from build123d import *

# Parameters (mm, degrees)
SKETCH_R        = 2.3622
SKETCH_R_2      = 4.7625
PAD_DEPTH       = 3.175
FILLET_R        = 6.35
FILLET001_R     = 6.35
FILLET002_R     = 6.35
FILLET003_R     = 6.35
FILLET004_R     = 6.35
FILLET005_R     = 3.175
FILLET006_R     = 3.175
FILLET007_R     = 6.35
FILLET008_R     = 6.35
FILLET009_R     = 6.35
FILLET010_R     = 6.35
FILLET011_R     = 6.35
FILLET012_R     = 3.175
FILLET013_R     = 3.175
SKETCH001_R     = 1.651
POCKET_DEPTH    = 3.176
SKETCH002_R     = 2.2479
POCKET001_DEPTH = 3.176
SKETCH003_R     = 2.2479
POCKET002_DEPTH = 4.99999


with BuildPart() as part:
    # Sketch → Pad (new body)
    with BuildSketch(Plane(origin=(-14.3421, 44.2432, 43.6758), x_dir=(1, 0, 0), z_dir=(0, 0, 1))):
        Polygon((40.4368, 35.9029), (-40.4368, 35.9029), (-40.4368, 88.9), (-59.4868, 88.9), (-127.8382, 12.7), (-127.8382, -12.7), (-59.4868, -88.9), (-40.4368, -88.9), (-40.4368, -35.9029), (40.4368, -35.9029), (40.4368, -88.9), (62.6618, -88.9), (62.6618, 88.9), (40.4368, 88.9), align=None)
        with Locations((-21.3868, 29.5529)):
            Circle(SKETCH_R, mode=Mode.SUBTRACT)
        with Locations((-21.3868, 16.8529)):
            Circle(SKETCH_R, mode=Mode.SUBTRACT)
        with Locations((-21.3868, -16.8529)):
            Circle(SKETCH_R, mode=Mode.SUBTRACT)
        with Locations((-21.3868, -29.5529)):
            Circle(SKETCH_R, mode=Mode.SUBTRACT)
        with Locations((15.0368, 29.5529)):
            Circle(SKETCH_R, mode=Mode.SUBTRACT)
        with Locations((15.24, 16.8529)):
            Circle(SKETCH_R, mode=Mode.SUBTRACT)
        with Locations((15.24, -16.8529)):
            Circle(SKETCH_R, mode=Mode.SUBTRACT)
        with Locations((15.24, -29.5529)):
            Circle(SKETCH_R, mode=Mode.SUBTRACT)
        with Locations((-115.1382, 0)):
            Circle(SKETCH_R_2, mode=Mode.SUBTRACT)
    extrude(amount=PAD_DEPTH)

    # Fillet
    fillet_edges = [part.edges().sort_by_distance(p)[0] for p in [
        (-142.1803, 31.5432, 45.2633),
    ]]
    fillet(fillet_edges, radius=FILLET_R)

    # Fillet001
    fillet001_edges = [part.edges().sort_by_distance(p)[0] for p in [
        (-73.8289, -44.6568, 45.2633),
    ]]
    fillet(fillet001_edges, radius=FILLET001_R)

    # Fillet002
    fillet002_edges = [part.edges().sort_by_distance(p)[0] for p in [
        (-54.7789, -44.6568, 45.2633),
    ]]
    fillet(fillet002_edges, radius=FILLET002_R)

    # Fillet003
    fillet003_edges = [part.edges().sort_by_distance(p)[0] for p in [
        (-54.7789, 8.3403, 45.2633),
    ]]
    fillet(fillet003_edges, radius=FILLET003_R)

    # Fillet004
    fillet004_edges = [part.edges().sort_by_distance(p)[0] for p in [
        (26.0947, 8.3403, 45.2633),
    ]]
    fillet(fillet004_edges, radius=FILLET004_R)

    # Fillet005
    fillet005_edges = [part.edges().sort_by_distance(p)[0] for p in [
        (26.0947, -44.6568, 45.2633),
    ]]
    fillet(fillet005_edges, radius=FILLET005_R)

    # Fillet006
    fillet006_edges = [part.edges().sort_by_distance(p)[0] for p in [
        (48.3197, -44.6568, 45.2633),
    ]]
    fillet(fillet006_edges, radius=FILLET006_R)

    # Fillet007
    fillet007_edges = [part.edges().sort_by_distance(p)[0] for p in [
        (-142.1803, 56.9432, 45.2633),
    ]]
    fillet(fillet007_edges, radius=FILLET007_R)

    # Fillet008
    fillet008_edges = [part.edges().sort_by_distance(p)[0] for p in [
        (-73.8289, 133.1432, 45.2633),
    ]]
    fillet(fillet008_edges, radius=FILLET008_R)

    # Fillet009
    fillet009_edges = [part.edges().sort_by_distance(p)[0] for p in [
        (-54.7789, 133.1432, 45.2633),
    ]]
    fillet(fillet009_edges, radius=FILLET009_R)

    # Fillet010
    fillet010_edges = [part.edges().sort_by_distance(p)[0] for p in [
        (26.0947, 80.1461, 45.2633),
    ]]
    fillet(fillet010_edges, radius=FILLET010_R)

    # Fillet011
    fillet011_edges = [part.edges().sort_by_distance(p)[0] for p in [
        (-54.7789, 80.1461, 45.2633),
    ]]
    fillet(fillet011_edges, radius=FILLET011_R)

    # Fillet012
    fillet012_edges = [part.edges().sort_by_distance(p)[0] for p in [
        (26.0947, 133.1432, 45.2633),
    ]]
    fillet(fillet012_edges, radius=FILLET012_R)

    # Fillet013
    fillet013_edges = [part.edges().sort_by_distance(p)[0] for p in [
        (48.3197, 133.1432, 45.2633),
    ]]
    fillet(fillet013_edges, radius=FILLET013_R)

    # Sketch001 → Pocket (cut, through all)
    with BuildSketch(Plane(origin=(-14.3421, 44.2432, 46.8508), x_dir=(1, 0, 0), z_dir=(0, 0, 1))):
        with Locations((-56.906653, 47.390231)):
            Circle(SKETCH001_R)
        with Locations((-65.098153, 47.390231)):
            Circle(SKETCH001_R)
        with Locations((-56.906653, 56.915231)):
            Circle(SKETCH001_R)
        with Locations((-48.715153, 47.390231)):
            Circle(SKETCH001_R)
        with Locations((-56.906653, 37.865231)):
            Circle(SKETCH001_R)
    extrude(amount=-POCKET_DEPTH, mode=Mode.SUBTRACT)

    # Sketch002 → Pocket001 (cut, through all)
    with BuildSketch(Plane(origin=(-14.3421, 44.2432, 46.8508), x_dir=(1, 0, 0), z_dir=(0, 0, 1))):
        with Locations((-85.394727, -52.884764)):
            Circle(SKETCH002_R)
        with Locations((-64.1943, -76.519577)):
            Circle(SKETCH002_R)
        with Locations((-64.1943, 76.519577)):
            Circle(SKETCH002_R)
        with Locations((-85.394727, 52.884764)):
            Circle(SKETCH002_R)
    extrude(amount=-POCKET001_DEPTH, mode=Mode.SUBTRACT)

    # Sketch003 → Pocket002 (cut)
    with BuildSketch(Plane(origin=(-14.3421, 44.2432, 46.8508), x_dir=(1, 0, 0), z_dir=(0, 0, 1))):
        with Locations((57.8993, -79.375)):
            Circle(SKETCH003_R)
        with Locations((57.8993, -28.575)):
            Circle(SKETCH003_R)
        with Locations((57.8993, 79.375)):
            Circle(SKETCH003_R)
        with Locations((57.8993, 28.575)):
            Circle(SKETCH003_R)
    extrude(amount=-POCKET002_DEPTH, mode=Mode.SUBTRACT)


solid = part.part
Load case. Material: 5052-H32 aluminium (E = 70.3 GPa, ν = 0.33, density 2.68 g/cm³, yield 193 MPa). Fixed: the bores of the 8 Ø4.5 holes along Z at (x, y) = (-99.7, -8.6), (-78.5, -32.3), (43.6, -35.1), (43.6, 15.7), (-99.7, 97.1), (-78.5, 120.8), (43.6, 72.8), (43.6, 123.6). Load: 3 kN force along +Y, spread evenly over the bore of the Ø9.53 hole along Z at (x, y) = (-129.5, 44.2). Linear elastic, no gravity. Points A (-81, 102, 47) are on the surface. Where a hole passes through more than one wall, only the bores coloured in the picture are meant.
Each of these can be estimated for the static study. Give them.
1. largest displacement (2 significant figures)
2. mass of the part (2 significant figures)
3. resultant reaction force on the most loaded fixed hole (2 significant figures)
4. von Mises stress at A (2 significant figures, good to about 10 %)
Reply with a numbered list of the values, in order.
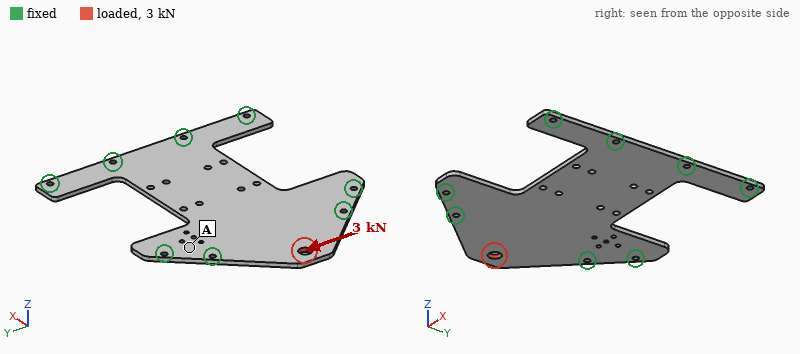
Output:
1. 29 µm
2. 170 g
3. 1.5 kN
4. 7.3 MPa
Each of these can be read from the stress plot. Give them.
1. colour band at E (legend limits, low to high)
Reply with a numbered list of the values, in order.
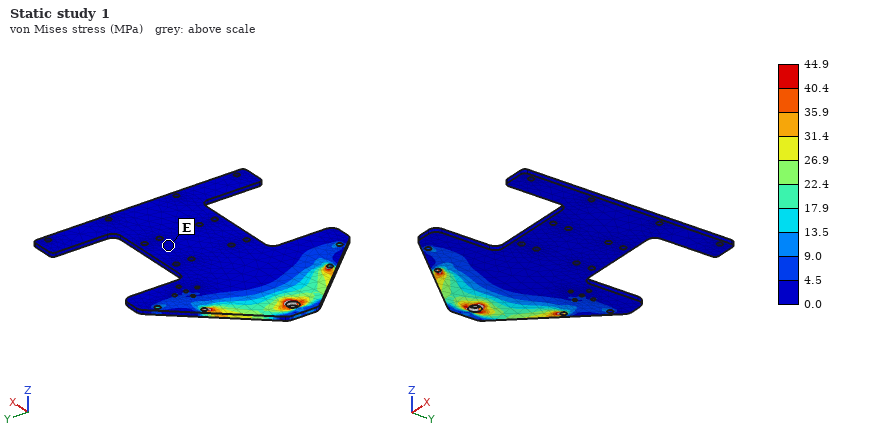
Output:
1. 0.0 to 4.5 MPa
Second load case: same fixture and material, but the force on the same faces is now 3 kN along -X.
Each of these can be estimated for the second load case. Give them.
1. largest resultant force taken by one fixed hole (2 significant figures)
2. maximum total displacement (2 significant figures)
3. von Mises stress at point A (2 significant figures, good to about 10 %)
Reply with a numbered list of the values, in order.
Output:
1. 1.0 kN
2. 28 µm
3. 6.8 MPa
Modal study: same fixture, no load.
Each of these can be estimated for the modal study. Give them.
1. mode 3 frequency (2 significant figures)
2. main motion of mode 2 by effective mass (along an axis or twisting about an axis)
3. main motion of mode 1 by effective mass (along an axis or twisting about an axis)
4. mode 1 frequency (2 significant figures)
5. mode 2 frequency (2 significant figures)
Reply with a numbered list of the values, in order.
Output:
1. 1600 Hz
2. along Z
3. along Z
4. 780 Hz
5. 1000 Hz
